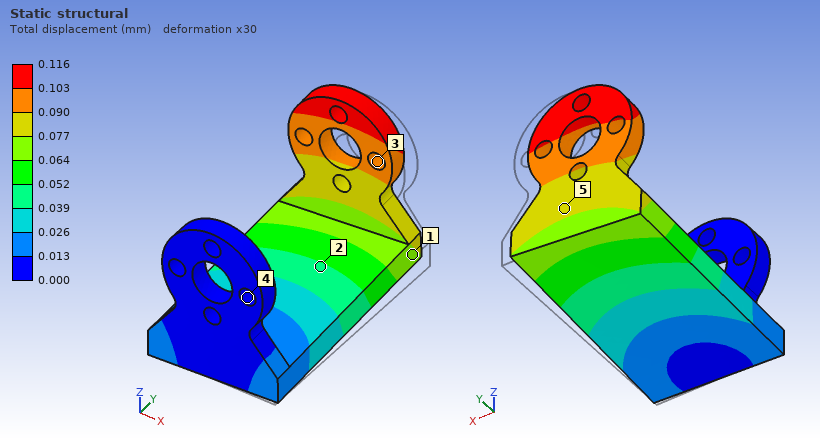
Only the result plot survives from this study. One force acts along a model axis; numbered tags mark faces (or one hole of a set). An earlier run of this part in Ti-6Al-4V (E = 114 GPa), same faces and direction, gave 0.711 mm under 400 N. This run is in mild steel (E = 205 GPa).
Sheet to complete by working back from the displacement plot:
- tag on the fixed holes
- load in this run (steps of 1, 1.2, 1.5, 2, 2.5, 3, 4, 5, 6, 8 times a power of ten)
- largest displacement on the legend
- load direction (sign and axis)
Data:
4
120 N
0.116 mm
-X
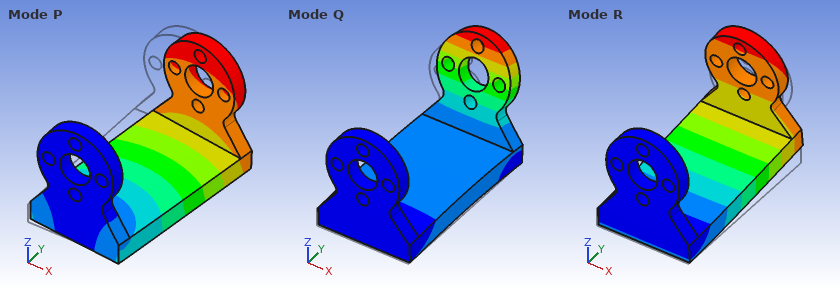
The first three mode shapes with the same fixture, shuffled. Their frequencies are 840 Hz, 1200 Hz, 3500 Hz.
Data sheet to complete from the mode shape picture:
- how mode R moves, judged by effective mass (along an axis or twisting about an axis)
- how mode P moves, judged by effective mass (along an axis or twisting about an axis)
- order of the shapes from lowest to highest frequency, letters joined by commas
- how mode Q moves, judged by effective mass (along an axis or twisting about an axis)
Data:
along Z
along X
R, P, Q
along Y
